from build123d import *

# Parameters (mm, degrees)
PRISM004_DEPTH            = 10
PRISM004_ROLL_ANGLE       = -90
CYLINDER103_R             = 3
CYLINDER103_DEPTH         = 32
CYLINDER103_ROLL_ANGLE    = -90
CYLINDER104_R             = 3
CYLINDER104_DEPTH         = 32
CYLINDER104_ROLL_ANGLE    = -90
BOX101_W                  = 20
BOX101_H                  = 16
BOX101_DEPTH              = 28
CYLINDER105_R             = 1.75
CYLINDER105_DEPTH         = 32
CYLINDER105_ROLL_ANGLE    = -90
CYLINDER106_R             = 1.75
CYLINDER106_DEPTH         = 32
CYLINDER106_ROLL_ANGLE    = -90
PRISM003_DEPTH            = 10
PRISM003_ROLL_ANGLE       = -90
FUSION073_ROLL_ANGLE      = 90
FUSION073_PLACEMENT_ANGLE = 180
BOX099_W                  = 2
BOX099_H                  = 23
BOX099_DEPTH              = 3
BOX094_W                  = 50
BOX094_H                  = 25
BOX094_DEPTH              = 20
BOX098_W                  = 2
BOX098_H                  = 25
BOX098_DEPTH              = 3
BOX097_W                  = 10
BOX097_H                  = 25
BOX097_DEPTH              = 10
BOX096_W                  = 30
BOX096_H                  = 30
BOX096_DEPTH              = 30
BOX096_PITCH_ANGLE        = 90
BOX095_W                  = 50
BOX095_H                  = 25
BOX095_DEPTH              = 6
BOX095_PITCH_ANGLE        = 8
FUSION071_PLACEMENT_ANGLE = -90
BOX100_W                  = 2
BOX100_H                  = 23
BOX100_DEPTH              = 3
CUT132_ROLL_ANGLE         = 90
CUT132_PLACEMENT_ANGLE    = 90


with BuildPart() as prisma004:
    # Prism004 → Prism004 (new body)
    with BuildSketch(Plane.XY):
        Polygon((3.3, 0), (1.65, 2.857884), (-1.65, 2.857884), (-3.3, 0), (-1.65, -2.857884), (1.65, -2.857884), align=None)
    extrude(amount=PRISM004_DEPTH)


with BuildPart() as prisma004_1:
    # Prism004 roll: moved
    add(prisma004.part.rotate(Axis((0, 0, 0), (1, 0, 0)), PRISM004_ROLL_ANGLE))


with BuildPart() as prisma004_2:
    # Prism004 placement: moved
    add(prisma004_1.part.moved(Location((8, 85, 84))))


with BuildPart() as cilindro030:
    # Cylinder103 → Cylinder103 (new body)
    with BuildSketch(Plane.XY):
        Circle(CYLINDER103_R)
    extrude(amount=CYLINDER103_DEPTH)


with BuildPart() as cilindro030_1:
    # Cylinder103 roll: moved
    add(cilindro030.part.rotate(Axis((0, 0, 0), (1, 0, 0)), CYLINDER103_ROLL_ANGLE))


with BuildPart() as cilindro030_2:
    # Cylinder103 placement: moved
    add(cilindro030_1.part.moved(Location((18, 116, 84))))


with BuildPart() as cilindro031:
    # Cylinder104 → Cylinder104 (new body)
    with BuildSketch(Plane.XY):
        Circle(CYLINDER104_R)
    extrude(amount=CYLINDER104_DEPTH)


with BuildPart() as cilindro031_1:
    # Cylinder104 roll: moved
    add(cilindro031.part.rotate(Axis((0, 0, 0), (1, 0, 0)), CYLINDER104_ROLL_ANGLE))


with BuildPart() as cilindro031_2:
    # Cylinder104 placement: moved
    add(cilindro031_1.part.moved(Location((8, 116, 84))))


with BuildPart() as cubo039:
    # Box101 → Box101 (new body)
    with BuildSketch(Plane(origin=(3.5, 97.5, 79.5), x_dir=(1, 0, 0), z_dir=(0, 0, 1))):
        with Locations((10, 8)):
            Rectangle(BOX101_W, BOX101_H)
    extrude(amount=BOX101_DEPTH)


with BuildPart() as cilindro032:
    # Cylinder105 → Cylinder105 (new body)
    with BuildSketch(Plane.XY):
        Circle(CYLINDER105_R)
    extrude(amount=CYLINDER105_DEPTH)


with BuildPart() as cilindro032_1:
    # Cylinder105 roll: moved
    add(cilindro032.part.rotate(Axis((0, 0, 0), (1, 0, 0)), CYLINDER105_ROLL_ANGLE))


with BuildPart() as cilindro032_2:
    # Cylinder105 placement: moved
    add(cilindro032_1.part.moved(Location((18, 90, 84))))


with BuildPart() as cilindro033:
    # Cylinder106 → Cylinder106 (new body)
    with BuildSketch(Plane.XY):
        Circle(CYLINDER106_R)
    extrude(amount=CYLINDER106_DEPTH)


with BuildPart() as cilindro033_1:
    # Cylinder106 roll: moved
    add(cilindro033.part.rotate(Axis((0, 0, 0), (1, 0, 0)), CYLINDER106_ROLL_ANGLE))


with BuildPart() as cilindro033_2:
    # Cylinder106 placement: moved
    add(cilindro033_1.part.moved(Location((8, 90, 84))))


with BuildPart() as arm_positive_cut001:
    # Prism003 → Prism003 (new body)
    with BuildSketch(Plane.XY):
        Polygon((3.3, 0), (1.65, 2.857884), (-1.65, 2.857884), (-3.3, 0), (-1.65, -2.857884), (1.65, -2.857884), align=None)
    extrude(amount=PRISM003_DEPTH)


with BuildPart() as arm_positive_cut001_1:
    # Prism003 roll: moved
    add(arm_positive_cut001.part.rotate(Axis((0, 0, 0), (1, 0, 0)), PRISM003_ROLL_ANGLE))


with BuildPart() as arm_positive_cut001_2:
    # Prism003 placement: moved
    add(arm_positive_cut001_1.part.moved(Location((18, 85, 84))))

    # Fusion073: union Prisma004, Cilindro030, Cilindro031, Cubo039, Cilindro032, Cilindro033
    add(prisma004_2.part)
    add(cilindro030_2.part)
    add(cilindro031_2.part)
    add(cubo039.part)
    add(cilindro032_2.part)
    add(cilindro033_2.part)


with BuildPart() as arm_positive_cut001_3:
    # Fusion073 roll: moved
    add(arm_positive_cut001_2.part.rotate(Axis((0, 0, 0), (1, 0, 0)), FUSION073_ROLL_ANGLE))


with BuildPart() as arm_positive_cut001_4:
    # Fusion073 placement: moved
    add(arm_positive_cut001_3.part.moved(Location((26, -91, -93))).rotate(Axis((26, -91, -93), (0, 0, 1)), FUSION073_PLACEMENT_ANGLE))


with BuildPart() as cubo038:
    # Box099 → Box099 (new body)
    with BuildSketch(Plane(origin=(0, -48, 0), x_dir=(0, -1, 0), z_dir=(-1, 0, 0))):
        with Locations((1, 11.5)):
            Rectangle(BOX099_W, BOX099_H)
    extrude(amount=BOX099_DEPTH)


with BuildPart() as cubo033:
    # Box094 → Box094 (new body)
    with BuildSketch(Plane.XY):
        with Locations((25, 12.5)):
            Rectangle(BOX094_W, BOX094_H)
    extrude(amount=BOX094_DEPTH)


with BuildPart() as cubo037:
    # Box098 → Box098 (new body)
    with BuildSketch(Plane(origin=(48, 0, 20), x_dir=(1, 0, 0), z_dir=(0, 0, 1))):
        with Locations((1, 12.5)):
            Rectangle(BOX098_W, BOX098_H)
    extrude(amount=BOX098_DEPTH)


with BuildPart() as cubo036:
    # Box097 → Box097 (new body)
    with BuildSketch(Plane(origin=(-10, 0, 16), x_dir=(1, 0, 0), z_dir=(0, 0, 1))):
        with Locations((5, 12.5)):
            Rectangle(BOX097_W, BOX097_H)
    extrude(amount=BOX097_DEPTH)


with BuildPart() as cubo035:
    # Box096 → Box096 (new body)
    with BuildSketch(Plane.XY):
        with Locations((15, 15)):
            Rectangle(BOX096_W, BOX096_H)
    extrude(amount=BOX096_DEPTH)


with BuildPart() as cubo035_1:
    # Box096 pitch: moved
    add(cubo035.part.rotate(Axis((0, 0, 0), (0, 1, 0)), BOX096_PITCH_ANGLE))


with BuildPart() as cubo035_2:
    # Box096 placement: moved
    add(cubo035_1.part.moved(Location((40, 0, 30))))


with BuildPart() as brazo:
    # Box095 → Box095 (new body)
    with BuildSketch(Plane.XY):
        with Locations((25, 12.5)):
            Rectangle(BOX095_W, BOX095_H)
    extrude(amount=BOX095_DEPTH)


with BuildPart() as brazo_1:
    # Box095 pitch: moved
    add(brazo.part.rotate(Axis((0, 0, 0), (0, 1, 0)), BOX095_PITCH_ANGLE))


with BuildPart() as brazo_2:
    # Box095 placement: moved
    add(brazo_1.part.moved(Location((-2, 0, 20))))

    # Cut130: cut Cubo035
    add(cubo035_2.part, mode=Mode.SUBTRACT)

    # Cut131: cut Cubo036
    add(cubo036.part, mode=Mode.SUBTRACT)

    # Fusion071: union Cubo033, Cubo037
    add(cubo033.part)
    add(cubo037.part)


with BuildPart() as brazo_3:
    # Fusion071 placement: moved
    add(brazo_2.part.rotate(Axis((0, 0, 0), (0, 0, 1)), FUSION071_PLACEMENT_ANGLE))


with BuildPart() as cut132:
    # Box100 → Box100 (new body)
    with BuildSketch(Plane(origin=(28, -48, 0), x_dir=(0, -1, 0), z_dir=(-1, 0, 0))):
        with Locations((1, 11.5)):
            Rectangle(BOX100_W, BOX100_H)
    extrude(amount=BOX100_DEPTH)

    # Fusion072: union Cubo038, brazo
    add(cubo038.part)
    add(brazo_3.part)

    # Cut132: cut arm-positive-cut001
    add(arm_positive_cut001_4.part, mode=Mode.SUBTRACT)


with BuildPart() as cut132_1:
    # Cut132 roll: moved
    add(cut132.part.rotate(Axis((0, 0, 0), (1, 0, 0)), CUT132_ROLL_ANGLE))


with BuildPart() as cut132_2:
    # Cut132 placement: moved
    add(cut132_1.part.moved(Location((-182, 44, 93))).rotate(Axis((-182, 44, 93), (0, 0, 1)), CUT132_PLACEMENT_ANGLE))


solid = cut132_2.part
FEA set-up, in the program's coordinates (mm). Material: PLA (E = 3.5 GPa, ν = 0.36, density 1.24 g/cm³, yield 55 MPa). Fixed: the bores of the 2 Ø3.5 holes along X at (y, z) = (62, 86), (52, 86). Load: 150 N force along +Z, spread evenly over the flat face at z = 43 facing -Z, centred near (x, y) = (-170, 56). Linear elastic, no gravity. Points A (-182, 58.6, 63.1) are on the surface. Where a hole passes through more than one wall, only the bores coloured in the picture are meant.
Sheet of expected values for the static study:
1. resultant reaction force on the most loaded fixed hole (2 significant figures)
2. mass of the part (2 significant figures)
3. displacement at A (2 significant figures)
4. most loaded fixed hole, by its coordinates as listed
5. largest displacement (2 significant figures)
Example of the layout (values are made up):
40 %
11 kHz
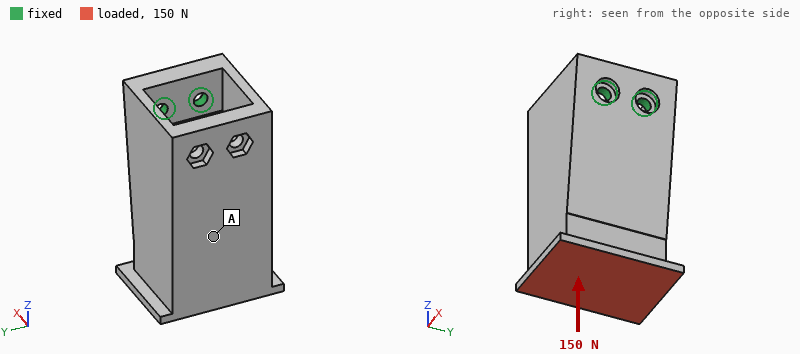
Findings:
87 N
30 g
0.48 mm
(52, 86)
0.73 mm
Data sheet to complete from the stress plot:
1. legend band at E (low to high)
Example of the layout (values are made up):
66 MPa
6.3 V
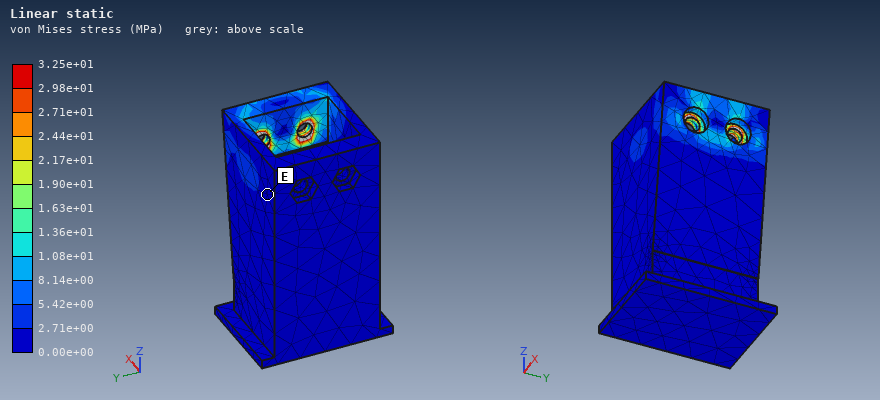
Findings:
0.00e+00 to 2.71e+00 MPa
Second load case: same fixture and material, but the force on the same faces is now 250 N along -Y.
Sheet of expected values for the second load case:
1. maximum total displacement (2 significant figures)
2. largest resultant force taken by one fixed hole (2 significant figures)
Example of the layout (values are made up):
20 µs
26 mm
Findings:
0.58 mm
900 N
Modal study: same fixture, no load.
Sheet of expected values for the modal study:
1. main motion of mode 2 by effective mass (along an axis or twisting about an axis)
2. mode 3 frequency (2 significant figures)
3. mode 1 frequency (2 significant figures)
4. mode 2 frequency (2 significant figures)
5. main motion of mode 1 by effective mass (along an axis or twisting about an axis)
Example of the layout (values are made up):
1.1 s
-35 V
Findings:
along Y
1700 Hz
350 Hz
1000 Hz
along X
